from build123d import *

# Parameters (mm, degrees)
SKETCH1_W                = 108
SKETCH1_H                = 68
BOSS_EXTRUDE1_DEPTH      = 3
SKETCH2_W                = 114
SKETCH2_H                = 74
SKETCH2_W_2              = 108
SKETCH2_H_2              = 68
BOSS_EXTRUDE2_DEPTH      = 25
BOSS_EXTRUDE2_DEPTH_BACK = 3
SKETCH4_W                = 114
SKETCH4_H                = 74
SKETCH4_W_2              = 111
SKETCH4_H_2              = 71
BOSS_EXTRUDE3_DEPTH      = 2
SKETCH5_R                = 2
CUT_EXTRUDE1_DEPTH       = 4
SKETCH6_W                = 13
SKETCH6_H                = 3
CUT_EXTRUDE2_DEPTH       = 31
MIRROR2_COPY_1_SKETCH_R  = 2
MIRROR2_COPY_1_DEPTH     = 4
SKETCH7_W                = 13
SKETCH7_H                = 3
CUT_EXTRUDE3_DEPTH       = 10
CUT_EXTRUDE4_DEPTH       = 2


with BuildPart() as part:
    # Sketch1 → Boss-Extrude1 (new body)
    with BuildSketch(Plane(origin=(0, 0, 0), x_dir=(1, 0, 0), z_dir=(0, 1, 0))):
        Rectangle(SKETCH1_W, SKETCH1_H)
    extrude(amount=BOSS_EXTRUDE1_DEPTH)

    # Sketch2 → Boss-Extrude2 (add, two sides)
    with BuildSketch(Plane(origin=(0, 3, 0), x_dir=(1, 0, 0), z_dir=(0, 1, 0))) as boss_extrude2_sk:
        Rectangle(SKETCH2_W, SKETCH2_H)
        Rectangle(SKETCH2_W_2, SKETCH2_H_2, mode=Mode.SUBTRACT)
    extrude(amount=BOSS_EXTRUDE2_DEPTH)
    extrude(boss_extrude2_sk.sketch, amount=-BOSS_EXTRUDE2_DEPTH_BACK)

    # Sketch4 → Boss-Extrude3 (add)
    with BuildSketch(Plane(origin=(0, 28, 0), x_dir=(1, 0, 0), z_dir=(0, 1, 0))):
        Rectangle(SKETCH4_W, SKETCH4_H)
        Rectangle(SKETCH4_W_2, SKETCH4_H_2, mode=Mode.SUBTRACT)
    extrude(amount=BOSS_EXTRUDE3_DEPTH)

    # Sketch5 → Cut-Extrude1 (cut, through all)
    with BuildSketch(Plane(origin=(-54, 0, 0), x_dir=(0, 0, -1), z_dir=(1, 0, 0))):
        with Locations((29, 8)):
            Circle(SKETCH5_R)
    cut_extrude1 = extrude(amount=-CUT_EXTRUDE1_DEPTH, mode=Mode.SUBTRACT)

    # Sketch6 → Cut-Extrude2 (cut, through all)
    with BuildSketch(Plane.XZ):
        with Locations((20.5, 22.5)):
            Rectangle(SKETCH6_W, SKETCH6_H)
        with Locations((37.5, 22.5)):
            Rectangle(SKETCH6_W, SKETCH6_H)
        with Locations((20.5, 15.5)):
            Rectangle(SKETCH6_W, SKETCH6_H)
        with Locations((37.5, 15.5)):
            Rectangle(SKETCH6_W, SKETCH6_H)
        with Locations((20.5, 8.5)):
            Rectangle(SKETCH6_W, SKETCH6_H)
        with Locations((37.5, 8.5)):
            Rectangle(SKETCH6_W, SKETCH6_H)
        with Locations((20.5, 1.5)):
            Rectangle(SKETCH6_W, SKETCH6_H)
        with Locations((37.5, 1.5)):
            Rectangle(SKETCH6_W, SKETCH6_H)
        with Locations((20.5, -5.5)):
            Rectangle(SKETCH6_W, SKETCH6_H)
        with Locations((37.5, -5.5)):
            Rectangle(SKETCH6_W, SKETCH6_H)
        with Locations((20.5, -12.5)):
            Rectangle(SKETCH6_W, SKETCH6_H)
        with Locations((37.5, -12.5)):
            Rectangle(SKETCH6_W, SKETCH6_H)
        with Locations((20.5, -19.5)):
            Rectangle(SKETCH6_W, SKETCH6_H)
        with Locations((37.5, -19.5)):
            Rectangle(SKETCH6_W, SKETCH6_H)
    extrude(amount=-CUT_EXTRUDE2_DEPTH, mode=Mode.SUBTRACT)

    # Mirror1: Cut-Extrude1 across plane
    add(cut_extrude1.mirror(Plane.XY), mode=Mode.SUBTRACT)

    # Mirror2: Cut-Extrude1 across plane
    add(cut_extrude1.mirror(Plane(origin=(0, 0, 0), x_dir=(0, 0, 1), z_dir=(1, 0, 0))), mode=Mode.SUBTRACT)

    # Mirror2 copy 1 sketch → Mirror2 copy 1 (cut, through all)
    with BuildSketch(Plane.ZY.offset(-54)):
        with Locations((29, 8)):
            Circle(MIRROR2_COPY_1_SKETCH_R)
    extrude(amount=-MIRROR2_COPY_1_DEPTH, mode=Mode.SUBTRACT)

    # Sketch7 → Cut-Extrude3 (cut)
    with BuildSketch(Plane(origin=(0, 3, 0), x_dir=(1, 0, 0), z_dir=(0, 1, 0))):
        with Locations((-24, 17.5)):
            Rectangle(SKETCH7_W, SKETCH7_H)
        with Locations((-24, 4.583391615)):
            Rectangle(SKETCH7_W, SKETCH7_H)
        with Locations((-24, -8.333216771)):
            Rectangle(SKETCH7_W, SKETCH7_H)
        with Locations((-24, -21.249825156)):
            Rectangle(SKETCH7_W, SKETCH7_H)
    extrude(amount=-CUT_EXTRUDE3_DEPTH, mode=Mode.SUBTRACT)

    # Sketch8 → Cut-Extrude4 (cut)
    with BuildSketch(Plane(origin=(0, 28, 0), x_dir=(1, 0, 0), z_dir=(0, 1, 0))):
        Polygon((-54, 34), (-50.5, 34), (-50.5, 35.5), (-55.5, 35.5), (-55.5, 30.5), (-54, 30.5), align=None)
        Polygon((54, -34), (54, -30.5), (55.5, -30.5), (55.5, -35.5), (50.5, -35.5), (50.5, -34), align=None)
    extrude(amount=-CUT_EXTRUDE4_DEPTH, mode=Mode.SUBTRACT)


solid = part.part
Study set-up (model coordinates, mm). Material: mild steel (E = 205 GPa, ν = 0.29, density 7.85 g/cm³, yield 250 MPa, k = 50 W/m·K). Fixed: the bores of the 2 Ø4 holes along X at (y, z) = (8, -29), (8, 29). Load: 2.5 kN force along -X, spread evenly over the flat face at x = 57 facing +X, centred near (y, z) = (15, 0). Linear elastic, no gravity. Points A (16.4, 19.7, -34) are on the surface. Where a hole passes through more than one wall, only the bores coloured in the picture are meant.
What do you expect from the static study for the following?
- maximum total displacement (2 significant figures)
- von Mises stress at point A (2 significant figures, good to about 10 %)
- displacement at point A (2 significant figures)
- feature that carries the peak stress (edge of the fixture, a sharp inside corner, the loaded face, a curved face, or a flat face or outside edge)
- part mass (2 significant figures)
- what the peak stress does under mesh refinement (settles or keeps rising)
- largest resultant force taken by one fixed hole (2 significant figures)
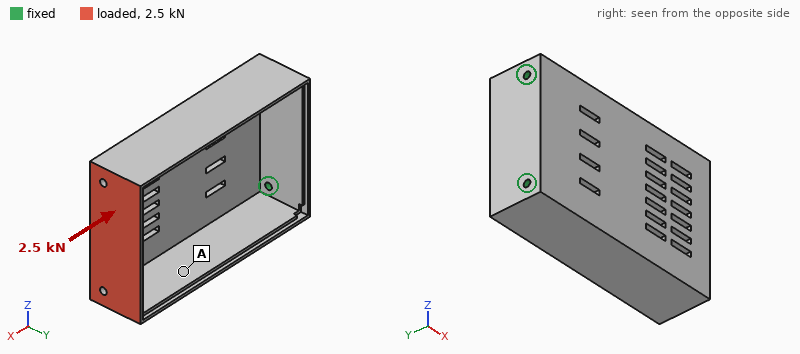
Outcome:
0.37 mm
15 MPa
0.18 mm
edge of the fixture
400 g
keeps rising
1.3 kN
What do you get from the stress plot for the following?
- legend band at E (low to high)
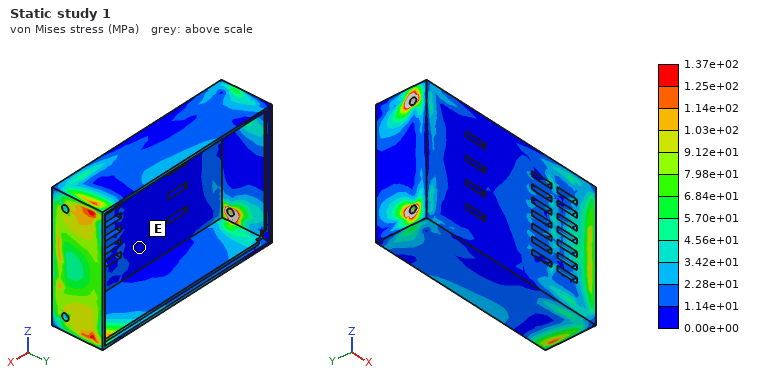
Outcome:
0.00e+00 to 1.14e+01 MPa
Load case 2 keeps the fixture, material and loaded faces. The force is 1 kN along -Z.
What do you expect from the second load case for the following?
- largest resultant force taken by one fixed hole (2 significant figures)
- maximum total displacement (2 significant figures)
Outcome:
1.9 kN
0.54 mm
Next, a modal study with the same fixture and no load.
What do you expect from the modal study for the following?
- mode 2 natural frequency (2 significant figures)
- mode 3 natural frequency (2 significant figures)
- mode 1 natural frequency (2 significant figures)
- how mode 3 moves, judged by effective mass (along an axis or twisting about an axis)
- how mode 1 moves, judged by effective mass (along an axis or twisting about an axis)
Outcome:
570 Hz
2000 Hz
340 Hz
along Z
along Y
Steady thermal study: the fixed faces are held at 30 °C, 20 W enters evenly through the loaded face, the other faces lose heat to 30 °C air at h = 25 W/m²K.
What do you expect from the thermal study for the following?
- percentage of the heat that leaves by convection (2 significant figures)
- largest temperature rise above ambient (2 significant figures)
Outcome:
86 %
65 K
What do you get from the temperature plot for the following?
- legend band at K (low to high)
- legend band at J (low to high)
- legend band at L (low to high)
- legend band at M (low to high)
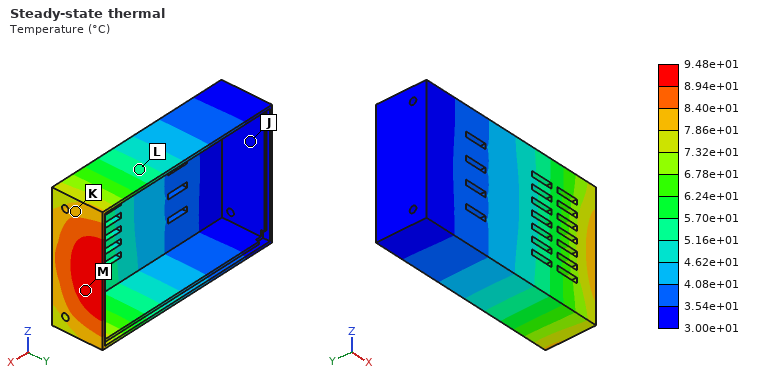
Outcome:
7.86e+01 to 8.40e+01 °C
3.00e+01 to 3.54e+01 °C
5.16e+01 to 5.70e+01 °C
8.94e+01 to 9.48e+01 °C
